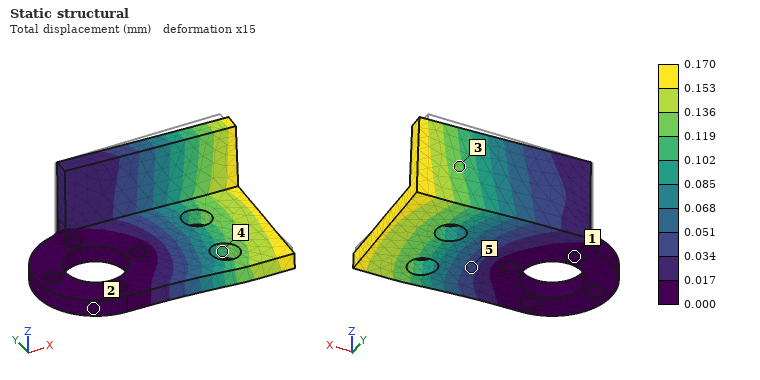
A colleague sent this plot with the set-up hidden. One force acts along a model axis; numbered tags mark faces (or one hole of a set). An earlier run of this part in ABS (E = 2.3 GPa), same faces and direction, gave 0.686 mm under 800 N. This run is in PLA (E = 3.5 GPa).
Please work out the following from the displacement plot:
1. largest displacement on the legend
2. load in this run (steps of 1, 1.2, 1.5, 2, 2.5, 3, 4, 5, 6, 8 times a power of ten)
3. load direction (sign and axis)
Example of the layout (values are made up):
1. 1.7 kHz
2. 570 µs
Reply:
1. 0.170 mm
2. 300 N
3. -Y
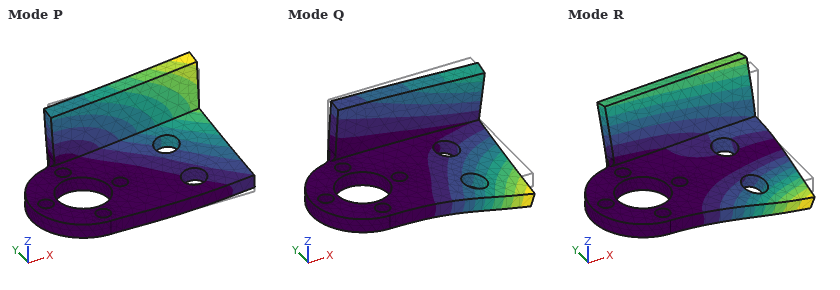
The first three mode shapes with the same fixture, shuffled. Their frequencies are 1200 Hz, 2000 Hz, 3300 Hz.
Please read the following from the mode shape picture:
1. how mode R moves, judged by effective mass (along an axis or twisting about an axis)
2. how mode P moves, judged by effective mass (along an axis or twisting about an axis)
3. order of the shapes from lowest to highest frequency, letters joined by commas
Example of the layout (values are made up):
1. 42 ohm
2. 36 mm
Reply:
1. along Y
2. along Z
3. P, Q, R
